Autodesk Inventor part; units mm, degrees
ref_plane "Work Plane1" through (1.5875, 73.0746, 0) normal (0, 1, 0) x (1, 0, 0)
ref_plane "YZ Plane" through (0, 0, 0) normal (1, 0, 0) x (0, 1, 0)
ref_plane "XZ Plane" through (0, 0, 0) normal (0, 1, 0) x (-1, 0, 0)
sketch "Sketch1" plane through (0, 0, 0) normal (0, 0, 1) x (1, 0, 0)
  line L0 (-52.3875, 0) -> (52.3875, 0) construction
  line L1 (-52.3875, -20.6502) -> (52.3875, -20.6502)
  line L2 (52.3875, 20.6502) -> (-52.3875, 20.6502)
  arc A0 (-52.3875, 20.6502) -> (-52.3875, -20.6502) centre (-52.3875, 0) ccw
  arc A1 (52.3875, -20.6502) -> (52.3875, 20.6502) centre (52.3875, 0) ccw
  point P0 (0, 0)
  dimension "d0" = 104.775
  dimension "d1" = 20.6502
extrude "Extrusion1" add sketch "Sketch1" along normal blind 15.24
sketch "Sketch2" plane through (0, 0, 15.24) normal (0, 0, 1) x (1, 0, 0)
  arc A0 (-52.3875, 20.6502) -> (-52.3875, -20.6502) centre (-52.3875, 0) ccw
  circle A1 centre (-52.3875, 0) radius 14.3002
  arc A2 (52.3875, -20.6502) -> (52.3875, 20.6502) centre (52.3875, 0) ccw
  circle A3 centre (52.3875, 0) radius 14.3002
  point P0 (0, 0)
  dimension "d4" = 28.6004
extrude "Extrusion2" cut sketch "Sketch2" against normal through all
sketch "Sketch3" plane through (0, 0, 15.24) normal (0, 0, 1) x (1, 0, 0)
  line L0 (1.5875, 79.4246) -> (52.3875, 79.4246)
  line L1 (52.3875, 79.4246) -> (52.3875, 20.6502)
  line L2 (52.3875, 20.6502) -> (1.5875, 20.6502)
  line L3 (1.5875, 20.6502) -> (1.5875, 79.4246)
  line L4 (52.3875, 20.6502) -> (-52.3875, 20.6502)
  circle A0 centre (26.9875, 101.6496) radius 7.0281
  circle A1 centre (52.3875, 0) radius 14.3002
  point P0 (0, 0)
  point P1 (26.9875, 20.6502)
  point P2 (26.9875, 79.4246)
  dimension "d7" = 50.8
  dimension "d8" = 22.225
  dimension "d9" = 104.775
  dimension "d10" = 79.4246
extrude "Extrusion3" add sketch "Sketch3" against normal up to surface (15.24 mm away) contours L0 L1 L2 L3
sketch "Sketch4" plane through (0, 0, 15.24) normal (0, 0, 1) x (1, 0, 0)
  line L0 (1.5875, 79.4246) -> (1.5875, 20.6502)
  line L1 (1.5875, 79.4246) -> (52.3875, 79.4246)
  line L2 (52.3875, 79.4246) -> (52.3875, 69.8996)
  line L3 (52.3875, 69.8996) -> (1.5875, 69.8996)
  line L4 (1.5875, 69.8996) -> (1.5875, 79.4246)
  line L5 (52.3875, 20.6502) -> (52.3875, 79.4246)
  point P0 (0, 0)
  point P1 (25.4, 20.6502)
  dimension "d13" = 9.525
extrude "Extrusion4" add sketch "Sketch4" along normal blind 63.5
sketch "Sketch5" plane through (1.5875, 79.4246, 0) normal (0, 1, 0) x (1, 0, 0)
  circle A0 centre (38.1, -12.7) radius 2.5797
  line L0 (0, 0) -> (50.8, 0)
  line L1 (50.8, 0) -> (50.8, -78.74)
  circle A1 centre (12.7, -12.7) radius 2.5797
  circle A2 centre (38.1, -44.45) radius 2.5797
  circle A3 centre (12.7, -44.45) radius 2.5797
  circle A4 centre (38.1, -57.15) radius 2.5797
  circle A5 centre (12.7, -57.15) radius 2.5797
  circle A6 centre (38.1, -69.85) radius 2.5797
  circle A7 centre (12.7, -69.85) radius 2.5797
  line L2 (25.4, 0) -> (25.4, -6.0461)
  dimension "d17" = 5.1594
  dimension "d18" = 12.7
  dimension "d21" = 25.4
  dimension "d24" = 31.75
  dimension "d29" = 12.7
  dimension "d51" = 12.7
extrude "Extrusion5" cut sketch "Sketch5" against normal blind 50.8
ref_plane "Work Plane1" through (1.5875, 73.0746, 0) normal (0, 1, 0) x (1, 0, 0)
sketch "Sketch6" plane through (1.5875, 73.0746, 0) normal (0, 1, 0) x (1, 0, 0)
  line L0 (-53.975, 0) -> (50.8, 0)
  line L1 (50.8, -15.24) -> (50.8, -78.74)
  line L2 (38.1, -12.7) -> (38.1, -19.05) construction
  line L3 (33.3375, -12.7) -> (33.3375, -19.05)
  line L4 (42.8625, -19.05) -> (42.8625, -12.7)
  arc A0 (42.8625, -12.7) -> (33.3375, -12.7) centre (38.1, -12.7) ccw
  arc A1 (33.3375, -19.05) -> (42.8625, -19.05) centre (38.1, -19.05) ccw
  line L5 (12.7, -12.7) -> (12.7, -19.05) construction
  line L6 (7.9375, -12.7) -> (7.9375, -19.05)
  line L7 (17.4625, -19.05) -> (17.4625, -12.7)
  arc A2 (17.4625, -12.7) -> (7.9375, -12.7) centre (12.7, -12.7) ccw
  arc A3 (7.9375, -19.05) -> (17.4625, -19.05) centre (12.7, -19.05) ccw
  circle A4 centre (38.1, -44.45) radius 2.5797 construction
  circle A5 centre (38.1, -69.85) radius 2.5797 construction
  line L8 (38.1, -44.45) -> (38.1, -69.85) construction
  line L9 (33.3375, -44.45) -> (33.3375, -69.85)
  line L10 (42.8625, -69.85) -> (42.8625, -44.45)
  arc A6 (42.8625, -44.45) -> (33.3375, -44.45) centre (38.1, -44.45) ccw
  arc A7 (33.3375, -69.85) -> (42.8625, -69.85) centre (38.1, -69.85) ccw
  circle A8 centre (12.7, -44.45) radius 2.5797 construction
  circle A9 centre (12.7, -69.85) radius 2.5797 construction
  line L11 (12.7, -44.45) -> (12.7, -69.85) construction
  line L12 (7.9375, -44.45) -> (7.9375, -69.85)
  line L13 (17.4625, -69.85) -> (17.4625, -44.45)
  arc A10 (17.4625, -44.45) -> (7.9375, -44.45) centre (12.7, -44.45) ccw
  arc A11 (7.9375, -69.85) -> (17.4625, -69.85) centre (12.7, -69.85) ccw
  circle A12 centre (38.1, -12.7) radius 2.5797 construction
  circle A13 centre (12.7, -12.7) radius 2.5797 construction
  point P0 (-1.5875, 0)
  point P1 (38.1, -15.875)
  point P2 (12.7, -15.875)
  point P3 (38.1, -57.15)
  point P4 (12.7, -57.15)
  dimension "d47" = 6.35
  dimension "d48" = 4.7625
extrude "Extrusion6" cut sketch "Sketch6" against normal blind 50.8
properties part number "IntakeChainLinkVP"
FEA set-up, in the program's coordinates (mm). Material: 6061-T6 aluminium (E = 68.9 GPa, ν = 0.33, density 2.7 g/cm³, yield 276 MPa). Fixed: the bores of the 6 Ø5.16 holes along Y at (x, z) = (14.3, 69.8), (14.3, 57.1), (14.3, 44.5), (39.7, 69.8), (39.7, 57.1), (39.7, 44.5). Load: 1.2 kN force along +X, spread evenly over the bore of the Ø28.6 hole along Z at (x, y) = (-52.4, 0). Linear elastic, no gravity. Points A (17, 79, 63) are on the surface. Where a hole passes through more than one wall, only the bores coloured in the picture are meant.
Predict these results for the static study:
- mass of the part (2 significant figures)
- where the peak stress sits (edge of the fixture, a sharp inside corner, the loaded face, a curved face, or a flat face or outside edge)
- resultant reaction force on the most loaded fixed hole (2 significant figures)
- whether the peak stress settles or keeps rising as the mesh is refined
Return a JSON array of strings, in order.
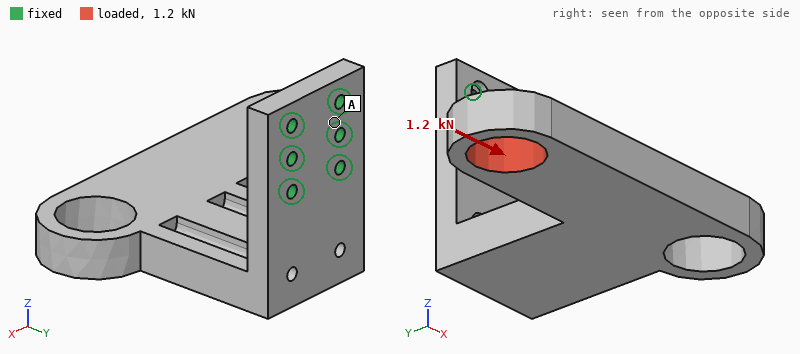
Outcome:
["360 g", "edge of the fixture", "3.7 kN", "keeps rising"]
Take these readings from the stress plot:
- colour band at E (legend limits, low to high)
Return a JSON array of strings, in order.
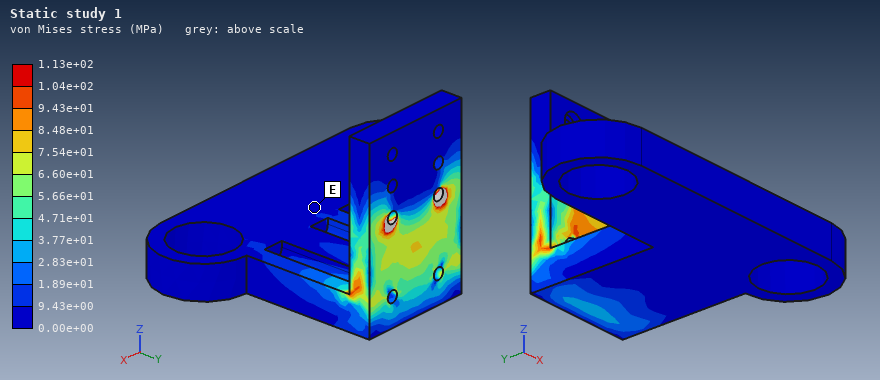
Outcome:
["0.00e+00 to 9.43e+00 MPa"]
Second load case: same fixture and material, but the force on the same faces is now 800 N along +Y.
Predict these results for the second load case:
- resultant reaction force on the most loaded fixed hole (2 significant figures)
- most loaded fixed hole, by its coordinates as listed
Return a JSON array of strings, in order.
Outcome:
["3.3 kN", "(14.3, 44.5)"]
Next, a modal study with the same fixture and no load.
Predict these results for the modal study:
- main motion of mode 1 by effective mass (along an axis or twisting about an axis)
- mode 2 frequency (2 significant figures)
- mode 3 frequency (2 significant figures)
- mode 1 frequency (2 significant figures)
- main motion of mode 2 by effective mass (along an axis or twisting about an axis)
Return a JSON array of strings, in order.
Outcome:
["along Z", "480 Hz", "1000 Hz", "320 Hz", "along X"]
